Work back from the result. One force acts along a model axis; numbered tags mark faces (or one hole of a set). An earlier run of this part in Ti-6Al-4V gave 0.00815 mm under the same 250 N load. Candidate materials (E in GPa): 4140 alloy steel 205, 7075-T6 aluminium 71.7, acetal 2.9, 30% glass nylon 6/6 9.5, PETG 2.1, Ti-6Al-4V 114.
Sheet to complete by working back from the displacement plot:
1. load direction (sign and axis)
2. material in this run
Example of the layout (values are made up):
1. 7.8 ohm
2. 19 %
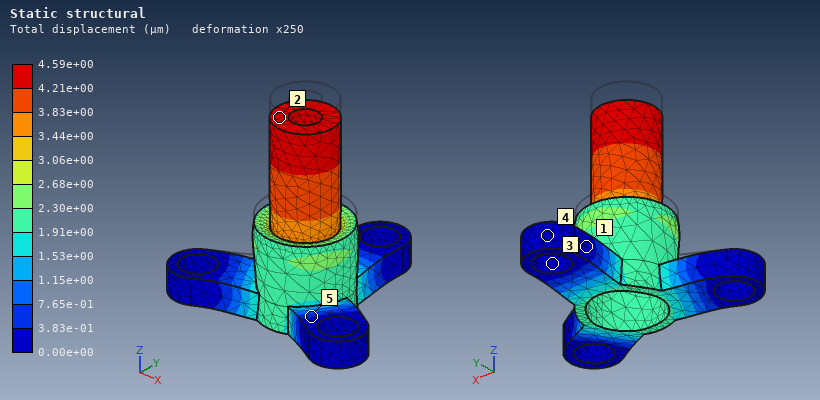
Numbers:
1. -Z
2. 4140 alloy steel
